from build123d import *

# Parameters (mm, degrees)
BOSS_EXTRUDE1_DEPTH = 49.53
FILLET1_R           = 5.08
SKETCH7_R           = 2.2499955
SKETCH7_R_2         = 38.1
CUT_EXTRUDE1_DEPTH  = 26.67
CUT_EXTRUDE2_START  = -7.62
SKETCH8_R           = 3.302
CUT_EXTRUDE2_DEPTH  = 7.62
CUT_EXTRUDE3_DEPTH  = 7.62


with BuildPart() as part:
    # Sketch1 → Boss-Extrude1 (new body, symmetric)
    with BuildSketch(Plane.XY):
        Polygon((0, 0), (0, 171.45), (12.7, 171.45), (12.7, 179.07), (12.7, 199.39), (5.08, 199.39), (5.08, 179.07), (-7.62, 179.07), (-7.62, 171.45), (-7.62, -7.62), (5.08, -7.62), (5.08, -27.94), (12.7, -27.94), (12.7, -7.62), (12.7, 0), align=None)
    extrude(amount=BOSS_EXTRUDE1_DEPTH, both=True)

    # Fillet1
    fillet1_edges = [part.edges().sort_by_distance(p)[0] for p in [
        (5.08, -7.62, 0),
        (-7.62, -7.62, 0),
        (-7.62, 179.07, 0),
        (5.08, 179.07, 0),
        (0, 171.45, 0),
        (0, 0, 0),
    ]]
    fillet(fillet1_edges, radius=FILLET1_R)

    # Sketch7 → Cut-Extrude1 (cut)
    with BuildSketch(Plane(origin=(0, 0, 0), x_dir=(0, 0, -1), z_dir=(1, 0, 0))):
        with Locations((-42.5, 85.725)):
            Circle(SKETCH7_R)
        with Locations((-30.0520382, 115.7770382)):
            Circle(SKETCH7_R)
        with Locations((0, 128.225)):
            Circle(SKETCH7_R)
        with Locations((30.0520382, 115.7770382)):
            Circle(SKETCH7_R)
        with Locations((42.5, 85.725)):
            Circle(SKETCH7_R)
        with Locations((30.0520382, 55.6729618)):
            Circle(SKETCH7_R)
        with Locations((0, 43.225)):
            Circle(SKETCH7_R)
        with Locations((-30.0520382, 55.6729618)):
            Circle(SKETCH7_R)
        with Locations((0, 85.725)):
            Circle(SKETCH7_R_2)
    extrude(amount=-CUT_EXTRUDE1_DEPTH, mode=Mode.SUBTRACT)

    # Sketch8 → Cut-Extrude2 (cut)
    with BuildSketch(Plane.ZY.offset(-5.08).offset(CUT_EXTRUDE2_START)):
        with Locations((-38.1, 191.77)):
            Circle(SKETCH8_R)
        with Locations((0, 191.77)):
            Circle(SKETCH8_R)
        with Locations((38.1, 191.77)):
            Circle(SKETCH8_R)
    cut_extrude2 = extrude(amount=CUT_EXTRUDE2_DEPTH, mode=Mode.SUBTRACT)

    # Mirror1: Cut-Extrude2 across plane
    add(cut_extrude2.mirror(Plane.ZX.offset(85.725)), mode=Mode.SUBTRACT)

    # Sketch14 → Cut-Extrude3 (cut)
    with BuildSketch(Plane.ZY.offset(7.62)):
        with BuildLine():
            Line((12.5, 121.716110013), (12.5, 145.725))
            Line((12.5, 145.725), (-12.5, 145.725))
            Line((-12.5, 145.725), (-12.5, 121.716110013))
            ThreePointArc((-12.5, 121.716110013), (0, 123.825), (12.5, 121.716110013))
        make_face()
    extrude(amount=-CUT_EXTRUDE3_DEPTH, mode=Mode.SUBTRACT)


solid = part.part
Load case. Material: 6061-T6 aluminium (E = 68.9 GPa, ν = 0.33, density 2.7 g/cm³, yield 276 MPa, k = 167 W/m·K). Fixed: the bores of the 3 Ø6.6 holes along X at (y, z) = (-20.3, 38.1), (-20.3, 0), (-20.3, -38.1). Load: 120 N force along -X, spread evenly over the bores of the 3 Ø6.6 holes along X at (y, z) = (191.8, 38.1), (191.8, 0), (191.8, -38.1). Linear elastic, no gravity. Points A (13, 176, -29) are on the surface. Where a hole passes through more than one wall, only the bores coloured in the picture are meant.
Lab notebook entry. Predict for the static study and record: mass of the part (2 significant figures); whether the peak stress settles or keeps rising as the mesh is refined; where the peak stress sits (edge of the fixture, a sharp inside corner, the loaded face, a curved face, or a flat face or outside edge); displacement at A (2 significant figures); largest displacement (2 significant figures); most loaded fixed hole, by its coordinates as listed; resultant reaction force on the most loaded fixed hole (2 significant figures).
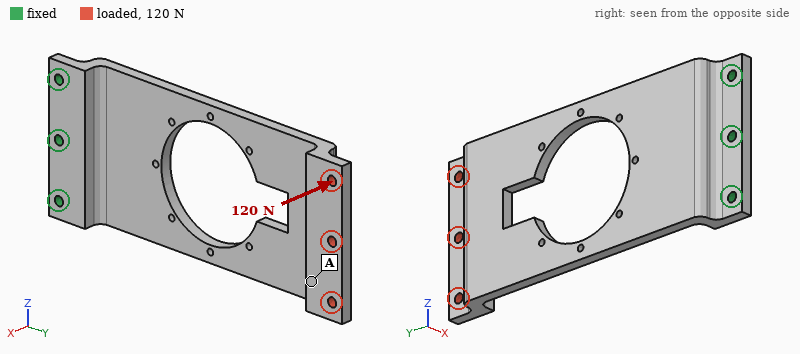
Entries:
410 g
keeps rising
a sharp inside corner
2.3 mm
2.8 mm
(-20.3, 0)
140 N
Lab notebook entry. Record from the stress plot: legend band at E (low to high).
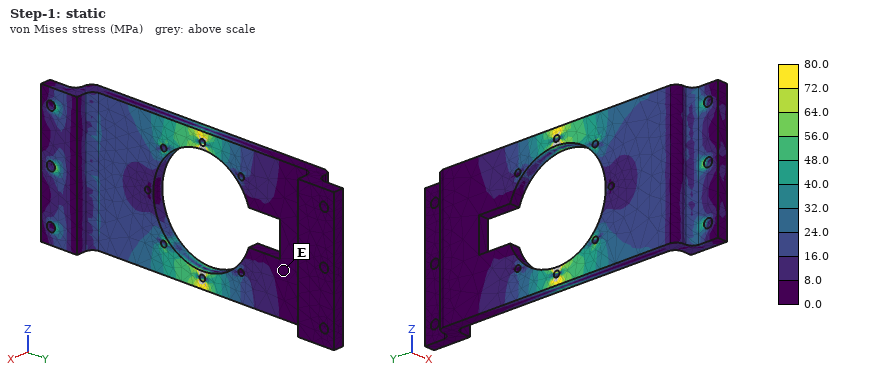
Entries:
0.0 to 8.0 MPa
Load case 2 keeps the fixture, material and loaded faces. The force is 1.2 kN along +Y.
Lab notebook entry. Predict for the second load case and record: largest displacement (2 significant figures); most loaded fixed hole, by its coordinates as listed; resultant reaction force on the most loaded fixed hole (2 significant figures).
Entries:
2.6 mm
(-20.3, 0)
450 N
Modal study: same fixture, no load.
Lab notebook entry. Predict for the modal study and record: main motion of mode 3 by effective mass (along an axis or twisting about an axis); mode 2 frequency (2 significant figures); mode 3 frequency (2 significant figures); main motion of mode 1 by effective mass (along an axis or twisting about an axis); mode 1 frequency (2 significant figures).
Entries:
along X
420 Hz
730 Hz
along X
100 Hz
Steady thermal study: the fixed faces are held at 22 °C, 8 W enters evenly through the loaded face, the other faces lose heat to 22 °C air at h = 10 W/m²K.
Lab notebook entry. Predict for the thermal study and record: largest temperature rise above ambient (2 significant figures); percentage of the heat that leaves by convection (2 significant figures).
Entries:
17 K
46 %
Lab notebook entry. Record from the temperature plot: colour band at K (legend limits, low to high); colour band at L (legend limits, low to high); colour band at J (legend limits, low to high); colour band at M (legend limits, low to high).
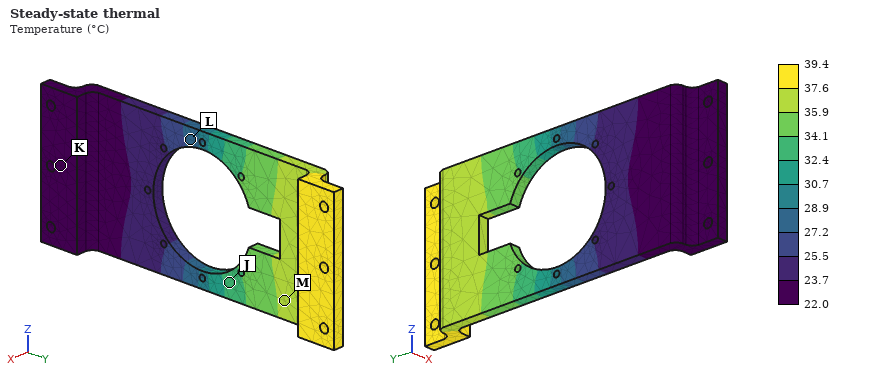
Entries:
22.0 to 23.7 °C
27.2 to 28.9 °C
32.4 to 34.1 °C
35.9 to 37.6 °C
